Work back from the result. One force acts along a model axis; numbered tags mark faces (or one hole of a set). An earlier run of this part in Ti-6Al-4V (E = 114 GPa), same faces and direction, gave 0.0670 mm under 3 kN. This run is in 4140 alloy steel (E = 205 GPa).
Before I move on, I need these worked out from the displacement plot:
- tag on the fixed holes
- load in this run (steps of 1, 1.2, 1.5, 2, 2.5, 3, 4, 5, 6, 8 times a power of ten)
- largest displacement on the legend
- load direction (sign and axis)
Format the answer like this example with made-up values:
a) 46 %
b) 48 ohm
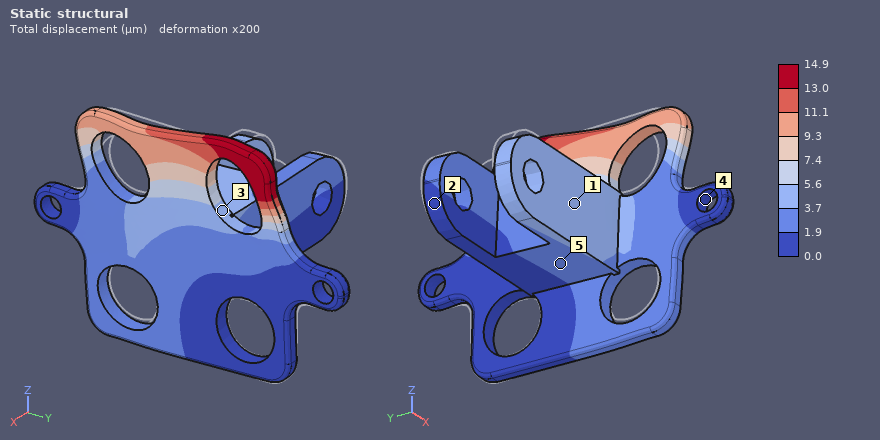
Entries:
a) 4
b) 1.2 kN
c) 14.9 µm
d) -Y
